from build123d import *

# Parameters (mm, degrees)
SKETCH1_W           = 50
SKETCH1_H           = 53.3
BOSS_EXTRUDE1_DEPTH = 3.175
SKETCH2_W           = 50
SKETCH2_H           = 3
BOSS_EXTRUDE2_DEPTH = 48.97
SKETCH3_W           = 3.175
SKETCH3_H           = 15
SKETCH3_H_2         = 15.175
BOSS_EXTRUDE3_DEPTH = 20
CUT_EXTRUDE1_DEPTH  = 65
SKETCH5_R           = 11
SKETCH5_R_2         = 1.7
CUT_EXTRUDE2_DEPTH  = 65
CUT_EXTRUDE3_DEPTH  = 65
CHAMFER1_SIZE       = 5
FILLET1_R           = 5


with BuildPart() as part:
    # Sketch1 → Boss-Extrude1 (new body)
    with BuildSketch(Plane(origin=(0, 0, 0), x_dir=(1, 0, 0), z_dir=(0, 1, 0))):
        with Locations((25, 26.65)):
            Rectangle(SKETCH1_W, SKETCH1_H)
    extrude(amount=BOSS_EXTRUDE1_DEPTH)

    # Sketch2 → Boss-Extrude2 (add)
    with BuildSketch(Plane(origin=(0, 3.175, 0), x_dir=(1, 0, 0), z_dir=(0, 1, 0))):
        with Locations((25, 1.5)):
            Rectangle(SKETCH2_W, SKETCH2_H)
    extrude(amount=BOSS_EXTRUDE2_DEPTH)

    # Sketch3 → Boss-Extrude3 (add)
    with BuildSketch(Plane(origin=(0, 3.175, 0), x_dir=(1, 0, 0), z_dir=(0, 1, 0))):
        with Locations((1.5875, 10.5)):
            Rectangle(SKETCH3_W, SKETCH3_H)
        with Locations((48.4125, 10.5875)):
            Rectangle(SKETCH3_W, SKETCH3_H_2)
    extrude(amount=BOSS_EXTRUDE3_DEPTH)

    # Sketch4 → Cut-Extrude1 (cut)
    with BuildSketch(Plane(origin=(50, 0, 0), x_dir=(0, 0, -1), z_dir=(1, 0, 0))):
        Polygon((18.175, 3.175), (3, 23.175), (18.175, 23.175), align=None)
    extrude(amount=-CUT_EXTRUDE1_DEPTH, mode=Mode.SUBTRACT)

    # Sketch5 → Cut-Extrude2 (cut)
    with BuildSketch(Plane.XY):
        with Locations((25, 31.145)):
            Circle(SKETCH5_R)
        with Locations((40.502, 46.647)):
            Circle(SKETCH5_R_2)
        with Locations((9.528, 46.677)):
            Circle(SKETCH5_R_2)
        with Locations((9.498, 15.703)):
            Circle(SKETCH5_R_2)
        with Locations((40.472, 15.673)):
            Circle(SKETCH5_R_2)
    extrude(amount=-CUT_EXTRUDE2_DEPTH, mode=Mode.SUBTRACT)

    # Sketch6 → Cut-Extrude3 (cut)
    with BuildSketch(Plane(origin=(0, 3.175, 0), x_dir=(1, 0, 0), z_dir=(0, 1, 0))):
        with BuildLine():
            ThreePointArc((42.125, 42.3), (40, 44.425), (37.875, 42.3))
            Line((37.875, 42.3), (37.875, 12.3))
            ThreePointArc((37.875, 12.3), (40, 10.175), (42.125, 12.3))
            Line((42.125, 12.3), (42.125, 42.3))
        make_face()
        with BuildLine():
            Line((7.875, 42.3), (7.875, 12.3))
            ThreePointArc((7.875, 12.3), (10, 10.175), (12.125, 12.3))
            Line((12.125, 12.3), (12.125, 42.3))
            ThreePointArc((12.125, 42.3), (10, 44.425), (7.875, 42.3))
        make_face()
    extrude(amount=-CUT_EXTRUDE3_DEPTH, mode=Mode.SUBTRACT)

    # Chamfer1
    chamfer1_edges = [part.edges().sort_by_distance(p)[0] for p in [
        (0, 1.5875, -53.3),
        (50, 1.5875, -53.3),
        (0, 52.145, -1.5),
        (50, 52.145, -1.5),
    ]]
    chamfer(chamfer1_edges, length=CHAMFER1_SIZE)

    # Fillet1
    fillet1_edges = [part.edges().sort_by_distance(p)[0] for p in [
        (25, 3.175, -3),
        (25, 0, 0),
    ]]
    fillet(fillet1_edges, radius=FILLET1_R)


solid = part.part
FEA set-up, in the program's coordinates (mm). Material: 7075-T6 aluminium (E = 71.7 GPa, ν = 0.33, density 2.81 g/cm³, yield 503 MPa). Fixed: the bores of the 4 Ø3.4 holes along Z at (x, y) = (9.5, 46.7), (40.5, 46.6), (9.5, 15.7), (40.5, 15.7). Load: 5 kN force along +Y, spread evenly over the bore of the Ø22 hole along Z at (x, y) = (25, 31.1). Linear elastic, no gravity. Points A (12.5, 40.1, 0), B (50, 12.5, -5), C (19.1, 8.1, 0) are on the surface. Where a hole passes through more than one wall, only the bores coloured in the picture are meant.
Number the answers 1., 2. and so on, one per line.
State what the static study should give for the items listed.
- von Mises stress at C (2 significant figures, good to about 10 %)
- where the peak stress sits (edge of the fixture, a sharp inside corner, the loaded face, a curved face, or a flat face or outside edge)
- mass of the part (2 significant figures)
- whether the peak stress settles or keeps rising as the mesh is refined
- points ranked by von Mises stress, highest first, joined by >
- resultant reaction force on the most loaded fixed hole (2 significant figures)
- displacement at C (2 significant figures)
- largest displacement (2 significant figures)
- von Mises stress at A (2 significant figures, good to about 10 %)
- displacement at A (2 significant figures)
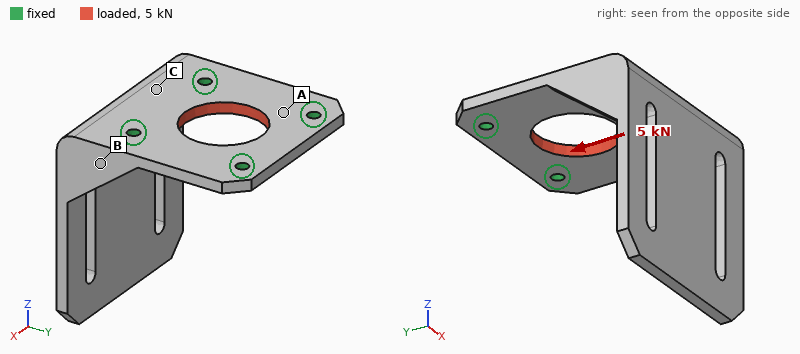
1. 15 MPa
2. edge of the fixture
3. 41 g
4. keeps rising
5. A > C > B
6. 1.3 kN
7. 5.0 µm
8. 15 µm
9. 36 MPa
10. 4.6 µm
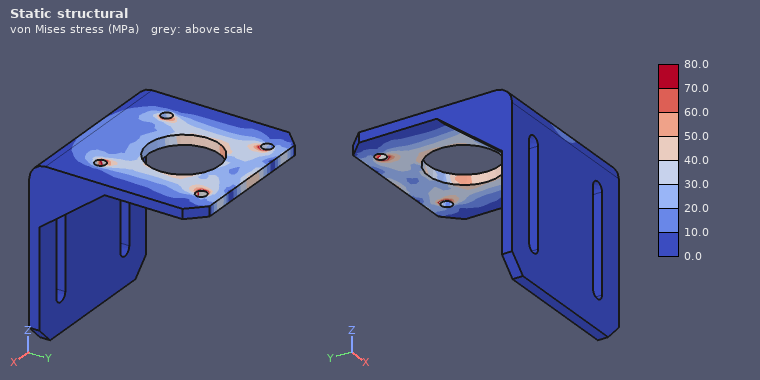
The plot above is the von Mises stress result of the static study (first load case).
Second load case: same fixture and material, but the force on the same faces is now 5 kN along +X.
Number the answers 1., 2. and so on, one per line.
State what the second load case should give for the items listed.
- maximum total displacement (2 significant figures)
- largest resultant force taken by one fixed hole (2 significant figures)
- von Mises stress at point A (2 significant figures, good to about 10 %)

1. 11 µm
2. 1.3 kN
3. 27 MPa
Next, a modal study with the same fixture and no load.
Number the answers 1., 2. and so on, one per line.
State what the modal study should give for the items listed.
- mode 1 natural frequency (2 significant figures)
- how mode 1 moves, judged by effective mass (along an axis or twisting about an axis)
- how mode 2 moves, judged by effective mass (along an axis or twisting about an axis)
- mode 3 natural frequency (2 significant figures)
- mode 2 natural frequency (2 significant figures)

1. 1000 Hz
2. along Y
3. along X
4. 3500 Hz
5. 2100 Hz
